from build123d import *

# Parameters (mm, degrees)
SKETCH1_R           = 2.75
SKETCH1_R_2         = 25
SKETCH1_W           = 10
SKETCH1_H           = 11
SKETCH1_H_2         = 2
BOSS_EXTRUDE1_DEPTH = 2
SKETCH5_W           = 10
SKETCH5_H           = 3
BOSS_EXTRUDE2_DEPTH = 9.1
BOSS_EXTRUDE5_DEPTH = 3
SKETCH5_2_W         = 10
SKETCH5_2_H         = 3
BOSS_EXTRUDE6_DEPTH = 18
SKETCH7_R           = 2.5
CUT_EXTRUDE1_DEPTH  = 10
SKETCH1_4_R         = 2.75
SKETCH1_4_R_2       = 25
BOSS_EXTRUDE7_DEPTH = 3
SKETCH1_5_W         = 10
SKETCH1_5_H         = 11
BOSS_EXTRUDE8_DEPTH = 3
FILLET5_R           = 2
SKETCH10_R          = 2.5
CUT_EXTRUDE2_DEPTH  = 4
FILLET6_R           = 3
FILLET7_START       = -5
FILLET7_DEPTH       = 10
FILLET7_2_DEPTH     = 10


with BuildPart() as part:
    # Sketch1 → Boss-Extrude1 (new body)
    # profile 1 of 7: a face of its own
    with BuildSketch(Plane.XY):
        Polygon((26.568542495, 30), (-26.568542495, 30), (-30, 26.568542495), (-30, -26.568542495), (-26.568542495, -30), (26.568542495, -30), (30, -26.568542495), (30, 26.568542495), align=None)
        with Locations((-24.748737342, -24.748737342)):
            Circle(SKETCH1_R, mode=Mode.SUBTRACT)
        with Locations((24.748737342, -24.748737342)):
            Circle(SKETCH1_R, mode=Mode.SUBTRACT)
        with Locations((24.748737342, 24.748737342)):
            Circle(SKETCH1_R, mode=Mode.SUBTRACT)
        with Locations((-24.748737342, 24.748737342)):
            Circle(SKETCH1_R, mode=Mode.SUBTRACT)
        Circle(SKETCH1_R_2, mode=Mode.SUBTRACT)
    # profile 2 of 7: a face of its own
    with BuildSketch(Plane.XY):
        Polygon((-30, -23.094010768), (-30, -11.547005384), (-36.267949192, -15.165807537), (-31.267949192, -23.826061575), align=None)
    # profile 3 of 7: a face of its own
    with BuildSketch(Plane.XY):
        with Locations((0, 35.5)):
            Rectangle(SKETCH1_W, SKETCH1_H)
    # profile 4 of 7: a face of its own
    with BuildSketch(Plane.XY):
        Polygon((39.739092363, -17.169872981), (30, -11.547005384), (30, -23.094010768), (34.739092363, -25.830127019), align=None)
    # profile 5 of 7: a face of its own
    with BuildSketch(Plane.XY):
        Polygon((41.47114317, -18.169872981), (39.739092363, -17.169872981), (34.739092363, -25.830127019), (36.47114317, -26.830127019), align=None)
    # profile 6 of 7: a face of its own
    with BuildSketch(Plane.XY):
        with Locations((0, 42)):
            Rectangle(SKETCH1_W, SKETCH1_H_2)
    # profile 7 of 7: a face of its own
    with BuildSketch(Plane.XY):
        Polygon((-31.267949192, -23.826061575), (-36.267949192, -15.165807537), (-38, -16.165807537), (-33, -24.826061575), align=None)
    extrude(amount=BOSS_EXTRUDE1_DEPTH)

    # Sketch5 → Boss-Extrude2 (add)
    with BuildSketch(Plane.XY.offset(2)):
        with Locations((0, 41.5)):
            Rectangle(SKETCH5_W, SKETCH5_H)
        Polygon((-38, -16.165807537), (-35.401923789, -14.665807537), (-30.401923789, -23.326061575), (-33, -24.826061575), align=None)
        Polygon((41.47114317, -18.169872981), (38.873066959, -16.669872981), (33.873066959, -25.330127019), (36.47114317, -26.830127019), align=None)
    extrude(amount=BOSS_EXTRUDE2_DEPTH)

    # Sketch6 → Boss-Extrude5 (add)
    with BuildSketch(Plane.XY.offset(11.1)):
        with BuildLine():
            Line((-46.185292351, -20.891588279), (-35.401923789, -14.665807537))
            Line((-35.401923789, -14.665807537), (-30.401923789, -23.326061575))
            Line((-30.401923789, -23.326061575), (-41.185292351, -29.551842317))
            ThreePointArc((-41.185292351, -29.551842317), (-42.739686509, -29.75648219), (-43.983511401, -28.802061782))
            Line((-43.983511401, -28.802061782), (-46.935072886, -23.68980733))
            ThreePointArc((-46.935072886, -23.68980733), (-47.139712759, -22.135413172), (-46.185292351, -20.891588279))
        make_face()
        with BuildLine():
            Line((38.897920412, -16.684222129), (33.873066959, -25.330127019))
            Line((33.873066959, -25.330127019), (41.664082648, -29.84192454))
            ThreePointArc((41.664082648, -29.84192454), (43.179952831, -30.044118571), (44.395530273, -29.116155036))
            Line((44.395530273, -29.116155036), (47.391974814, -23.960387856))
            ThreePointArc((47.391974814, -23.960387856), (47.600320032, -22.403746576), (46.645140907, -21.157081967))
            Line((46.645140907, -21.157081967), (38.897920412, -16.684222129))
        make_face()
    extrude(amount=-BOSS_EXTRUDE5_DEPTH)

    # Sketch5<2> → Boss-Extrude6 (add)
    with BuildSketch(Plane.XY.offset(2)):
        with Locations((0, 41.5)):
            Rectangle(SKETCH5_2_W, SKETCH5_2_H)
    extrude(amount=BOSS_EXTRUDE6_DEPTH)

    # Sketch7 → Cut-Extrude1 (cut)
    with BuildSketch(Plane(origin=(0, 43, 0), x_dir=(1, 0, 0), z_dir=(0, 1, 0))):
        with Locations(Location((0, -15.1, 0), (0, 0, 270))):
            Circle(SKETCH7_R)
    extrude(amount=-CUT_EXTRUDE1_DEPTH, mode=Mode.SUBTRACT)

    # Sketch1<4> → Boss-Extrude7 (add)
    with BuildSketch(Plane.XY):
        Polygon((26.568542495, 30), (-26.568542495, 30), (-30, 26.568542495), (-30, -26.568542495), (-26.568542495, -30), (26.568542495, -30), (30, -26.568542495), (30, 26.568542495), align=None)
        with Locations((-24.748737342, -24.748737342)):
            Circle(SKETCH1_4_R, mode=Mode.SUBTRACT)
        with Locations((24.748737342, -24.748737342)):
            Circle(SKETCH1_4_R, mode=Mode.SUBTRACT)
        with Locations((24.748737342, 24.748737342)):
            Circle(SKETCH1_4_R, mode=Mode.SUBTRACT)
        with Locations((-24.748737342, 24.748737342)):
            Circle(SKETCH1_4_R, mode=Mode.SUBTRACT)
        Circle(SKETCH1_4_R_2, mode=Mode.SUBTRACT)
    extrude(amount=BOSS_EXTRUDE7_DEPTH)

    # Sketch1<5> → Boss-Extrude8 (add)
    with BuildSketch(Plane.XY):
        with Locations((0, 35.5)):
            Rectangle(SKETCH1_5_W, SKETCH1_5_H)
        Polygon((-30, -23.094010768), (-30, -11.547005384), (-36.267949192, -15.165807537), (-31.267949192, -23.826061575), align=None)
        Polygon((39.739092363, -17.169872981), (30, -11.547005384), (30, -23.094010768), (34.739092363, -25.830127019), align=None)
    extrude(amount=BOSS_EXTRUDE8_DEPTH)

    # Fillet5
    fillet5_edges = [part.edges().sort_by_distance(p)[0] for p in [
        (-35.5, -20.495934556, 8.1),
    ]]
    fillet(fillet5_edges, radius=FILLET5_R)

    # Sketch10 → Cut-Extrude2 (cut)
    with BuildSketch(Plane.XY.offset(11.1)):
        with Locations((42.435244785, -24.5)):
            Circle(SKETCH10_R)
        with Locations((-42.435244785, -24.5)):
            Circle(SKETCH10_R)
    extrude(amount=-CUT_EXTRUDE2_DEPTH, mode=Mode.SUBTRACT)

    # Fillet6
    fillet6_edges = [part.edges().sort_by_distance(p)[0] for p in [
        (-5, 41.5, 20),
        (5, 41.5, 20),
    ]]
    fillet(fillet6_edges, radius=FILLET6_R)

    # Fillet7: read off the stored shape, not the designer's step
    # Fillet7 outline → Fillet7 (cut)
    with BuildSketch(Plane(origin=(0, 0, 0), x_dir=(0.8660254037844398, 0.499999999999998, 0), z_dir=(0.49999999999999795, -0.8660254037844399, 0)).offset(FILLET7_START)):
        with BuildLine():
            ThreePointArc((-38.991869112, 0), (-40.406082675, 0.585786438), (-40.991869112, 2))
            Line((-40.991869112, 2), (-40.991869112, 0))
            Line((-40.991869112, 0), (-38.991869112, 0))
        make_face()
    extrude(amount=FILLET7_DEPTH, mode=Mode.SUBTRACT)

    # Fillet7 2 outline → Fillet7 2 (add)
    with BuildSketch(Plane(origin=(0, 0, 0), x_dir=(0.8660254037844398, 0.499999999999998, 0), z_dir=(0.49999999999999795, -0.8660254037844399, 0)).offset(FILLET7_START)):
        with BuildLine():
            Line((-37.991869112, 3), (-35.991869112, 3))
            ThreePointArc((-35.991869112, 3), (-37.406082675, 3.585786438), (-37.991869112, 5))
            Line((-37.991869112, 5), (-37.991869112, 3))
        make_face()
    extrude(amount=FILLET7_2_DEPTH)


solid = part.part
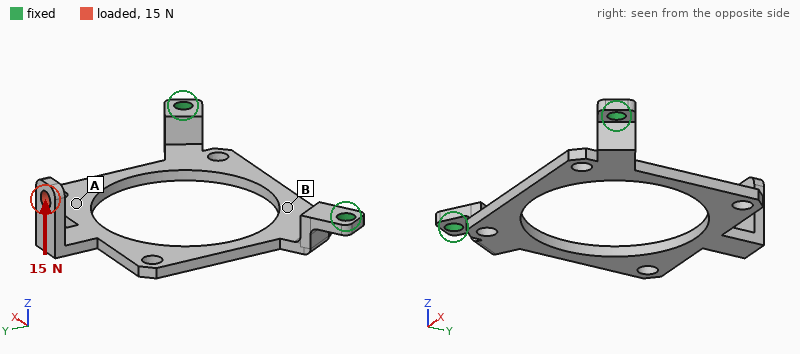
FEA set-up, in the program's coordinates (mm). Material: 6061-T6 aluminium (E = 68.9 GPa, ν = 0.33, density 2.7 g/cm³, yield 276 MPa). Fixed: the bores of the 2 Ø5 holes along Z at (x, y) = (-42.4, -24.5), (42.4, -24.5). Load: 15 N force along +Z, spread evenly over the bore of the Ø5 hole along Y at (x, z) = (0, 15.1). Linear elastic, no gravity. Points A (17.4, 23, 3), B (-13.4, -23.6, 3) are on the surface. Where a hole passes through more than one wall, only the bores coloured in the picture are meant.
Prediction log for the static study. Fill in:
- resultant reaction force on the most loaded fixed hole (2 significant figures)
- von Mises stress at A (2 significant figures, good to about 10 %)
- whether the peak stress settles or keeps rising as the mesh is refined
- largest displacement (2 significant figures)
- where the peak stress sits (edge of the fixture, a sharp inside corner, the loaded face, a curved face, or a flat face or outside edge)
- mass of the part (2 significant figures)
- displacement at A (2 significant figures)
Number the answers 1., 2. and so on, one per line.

1. 25 N
2. 10 MPa
3. keeps rising
4. 0.81 mm
5. a sharp inside corner
6. 18 g
7. 0.42 mm
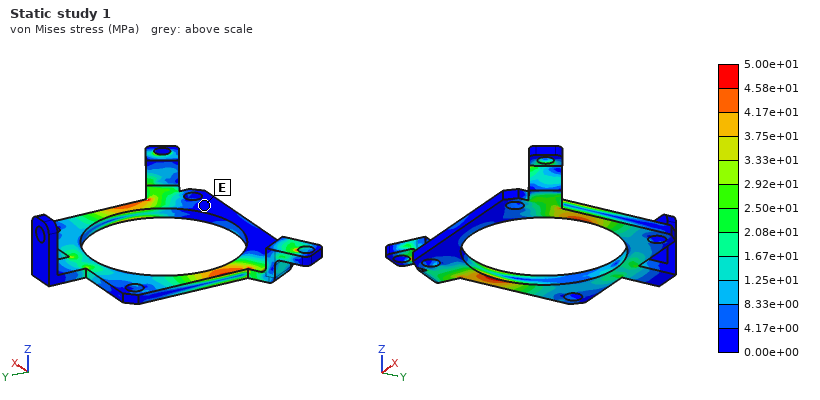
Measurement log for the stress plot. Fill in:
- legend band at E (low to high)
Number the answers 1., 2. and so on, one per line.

1. 0.00e+00 to 4.17e+00 MPa
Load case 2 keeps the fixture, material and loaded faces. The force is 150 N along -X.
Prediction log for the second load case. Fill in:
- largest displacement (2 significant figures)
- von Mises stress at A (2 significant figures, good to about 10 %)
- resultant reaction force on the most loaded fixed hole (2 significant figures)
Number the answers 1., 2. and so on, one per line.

1. 0.89 mm
2. 53 MPa
3. 150 N
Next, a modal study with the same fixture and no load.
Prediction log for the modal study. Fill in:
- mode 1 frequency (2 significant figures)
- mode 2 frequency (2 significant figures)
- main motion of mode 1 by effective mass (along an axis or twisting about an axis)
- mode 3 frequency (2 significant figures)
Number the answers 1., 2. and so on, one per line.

1. 370 Hz
2. 1300 Hz
3. along Z
4. 1900 Hz
